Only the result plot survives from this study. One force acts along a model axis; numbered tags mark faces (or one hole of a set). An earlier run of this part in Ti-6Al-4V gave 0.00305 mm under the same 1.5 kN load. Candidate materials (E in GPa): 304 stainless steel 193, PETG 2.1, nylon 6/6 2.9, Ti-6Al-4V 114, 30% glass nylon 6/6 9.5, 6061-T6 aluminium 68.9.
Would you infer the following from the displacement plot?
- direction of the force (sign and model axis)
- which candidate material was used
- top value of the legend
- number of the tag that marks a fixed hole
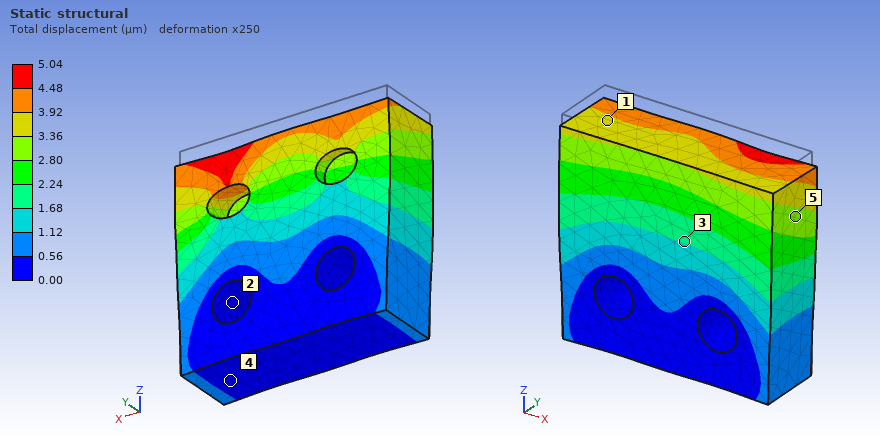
-Z
6061-T6 aluminium
5.04 µm
2
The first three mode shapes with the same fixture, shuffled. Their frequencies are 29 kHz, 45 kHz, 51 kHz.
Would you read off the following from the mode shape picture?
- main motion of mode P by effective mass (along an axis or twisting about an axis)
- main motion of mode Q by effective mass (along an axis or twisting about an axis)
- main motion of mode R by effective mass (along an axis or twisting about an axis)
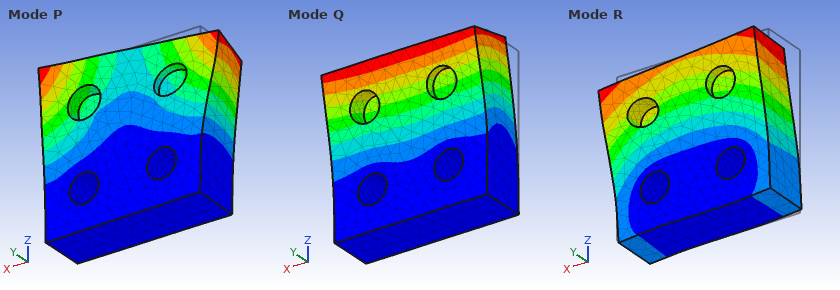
twisting about Z
along Y
along X
